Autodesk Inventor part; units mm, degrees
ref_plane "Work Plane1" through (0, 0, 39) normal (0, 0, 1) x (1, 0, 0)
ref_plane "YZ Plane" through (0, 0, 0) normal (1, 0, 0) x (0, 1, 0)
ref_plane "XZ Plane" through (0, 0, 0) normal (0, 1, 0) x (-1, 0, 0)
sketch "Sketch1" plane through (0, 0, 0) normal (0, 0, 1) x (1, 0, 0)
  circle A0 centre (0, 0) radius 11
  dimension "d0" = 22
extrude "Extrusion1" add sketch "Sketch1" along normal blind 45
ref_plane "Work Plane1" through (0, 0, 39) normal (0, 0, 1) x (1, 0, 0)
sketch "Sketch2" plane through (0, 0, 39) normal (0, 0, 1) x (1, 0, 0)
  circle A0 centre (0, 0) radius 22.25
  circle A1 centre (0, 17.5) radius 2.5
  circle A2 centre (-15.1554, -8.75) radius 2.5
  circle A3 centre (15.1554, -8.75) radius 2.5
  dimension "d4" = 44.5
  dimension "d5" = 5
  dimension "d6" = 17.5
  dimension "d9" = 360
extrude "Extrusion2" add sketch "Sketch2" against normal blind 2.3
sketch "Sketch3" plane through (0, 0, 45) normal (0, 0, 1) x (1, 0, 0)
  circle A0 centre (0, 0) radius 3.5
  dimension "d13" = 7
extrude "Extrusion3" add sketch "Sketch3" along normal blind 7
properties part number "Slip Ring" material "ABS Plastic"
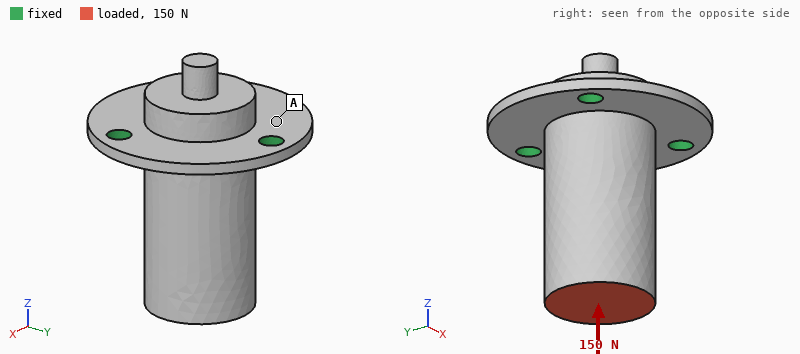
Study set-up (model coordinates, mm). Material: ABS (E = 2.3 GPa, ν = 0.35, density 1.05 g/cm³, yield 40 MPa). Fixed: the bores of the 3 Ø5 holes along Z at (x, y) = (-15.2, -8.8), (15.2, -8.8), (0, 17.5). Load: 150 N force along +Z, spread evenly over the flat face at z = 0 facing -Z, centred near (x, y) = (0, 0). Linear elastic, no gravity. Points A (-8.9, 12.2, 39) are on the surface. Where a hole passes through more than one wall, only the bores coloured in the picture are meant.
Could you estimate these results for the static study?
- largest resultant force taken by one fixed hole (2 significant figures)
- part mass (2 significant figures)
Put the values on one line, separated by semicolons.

50 N; 21 g
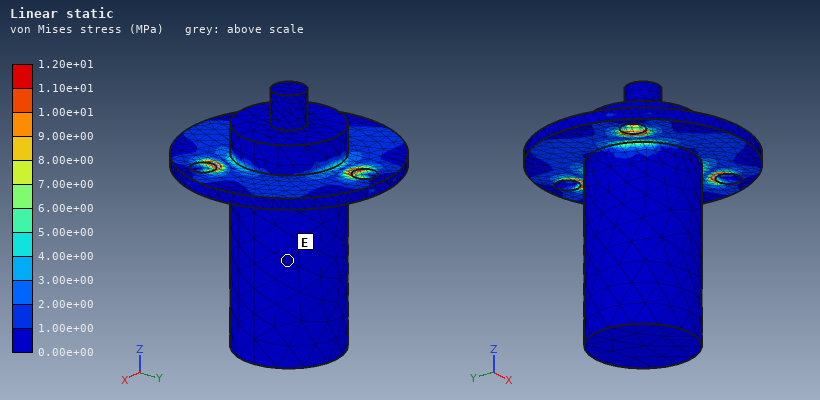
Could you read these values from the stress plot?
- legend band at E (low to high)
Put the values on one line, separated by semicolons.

0.00e+00 to 1.00e+00 MPa
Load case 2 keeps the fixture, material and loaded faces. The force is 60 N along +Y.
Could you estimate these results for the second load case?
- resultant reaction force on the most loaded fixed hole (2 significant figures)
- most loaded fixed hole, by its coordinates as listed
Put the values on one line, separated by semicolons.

100 N; (0, 17.5)
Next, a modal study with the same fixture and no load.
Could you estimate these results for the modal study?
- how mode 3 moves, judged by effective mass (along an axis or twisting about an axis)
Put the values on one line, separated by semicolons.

along Z
